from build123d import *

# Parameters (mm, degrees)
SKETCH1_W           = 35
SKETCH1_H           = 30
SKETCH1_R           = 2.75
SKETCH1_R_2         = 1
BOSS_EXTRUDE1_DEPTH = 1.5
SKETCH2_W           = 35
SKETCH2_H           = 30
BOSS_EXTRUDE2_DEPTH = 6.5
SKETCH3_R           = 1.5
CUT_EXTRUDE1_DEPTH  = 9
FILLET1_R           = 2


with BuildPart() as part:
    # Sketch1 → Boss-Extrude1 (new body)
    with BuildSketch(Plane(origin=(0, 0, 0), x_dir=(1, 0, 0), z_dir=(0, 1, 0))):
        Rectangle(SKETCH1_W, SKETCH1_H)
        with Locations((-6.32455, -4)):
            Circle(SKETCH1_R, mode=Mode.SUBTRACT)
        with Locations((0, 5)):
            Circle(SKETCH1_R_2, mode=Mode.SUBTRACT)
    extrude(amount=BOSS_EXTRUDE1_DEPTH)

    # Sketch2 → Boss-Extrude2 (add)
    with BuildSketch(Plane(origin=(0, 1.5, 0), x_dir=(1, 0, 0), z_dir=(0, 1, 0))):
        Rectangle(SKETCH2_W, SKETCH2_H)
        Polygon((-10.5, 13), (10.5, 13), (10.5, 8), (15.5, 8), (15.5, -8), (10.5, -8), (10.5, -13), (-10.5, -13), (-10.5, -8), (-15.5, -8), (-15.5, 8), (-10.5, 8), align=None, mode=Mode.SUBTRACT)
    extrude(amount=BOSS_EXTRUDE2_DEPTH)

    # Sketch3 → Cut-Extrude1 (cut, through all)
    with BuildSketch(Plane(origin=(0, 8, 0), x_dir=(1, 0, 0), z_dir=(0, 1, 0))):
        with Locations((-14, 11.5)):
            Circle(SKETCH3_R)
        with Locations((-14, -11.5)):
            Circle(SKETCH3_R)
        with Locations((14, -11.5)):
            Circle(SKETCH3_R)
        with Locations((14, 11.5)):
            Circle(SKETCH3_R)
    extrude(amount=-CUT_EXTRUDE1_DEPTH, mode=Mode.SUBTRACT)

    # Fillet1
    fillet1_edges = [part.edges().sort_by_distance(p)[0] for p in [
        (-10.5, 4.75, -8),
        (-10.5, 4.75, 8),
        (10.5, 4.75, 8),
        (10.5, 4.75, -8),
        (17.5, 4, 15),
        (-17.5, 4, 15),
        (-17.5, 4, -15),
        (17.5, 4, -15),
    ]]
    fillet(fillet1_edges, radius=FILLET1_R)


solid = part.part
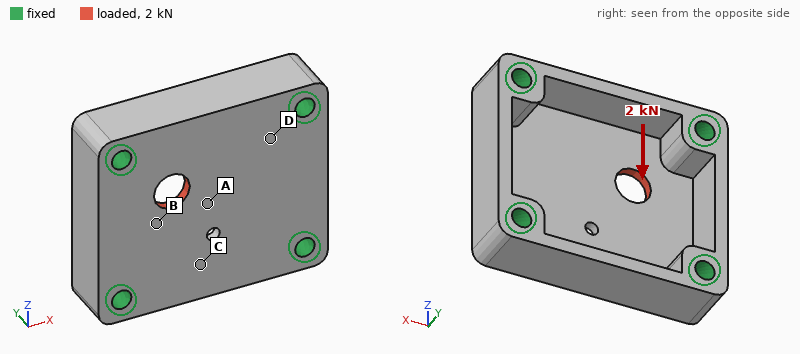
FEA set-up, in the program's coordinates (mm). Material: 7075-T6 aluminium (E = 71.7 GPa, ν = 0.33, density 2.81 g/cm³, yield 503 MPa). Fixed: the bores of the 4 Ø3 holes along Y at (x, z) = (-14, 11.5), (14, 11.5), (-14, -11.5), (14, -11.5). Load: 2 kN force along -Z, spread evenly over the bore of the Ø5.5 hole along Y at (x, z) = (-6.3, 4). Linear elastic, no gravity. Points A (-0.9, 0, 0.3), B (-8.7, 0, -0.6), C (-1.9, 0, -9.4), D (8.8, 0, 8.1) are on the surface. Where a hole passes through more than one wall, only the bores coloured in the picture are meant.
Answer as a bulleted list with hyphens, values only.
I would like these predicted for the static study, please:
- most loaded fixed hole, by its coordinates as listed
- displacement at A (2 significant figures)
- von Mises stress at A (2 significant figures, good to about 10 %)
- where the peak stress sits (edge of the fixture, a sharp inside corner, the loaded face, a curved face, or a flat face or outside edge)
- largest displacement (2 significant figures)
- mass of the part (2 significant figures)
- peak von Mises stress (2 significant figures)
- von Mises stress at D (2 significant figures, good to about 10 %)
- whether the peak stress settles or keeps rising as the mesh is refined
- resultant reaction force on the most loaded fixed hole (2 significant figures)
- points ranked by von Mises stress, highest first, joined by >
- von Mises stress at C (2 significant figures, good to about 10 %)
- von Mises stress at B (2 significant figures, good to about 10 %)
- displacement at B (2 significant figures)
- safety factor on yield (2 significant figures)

- (-14, 11.5)
- 8.4 µm
- 36 MPa
- the loaded face
- 15 µm
- 9.8 g
- 140 MPa
- 23 MPa
- settles
- 870 N
- B > A > D > C
- 11 MPa
- 61 MPa
- 7.3 µm
- 3.6
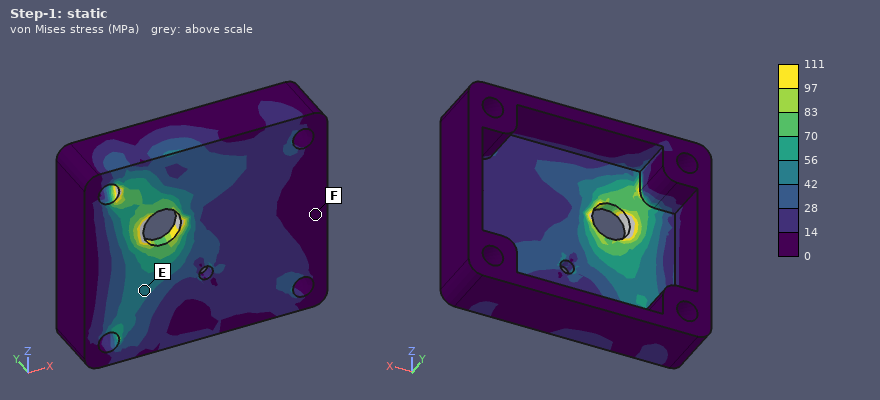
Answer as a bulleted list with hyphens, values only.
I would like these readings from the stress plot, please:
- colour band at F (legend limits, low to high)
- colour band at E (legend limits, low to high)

- 0 to 14 MPa
- 42 to 56 MPa
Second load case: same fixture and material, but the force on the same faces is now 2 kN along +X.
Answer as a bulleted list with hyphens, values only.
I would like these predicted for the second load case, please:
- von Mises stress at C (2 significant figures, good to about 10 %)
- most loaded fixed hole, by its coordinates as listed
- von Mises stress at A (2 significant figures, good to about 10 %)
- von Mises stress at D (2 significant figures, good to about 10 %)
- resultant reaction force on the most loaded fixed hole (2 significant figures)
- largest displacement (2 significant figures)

- 12 MPa
- (-14, 11.5)
- 50 MPa
- 31 MPa
- 880 N
- 13 µm
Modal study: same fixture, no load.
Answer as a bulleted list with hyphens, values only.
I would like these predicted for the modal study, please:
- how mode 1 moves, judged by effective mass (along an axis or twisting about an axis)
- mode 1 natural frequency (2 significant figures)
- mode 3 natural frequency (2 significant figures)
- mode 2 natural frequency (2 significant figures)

- along Y
- 14 kHz
- 28 kHz
- 26 kHz
